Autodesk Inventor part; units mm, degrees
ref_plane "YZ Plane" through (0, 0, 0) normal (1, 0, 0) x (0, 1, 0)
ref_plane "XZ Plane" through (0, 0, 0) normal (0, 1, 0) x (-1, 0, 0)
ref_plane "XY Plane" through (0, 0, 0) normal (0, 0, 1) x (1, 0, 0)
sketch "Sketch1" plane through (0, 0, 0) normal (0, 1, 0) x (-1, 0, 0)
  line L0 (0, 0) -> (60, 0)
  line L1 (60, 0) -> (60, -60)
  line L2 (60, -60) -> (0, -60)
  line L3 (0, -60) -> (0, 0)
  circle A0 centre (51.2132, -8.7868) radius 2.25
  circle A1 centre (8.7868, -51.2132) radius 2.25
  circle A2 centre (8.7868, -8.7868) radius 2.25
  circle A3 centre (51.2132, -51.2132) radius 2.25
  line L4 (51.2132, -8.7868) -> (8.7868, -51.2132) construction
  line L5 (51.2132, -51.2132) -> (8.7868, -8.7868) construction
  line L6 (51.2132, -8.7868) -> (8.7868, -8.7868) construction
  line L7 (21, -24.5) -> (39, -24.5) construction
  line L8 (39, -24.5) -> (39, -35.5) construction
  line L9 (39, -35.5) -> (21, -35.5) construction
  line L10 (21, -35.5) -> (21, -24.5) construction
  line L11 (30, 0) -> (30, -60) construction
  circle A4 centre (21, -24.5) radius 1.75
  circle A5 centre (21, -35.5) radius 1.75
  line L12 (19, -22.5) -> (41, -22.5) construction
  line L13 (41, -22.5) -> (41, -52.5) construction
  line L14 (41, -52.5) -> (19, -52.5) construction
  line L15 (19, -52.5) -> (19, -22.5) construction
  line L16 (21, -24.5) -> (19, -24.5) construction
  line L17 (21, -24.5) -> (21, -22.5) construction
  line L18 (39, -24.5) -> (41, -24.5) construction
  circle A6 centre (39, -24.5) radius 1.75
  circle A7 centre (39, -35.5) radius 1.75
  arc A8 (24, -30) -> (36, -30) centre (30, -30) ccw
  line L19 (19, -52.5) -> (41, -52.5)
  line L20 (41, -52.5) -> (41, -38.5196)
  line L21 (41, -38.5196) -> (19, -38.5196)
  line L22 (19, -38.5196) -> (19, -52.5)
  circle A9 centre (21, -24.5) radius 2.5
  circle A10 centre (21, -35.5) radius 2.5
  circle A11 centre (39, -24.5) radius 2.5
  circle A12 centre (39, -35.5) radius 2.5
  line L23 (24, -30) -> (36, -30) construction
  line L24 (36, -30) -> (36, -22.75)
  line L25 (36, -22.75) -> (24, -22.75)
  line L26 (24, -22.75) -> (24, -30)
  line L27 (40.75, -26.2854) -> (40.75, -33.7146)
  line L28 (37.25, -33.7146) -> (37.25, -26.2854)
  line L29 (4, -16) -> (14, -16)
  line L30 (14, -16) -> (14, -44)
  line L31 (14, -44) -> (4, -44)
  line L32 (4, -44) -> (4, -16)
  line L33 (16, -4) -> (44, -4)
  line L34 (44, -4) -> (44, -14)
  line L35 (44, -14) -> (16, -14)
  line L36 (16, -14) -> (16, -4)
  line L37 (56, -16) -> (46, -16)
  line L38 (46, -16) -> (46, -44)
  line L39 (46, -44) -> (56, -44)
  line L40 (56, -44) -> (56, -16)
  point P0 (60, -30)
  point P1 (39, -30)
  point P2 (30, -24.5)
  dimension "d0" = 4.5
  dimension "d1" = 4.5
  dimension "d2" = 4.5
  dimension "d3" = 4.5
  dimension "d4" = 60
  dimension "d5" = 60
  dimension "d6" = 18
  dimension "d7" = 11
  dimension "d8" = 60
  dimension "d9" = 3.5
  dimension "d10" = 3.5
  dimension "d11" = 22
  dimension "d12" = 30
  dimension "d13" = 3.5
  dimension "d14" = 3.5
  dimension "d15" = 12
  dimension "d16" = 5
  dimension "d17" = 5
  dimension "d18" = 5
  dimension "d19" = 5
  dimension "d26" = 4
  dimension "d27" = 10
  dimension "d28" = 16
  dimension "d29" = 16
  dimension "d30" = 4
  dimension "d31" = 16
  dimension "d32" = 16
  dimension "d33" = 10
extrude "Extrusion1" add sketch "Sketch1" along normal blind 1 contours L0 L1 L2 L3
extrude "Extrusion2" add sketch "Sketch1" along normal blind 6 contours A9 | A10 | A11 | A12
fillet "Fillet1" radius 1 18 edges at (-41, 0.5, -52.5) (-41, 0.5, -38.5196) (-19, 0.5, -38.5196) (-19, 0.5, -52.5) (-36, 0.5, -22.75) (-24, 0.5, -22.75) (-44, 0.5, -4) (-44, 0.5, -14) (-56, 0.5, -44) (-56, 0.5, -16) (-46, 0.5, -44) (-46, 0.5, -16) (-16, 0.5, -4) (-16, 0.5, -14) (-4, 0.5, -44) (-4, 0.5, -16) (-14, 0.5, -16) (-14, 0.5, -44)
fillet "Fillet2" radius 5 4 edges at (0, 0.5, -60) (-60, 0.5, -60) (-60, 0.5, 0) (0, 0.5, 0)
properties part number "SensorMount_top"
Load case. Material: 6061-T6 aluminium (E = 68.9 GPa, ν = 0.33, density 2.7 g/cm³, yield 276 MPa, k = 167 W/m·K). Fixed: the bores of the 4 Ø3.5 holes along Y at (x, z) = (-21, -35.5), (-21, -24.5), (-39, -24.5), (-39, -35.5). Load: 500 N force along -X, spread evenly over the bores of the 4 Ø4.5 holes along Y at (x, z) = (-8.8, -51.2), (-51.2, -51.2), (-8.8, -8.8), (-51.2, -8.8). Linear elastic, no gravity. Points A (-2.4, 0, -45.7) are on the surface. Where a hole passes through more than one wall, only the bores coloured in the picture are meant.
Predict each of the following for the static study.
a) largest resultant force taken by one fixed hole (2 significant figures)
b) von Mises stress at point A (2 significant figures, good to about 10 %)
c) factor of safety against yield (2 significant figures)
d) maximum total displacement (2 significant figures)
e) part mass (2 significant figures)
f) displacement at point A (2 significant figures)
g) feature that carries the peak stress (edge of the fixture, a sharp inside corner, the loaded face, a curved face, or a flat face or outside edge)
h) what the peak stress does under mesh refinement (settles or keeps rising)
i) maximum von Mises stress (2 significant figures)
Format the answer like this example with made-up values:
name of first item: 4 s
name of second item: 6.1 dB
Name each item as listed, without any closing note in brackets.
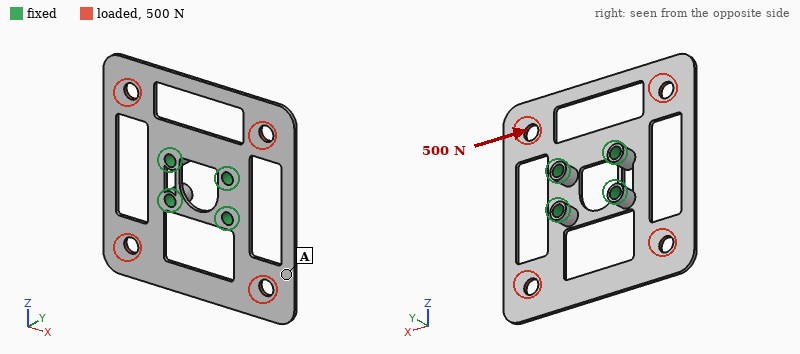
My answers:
largest resultant force taken by one fixed hole: 180 N
von Mises stress at point A: 14 MPa
factor of safety against yield: 1.1
maximum total displacement: 42 µm
part mass: 6.4 g
displacement at point A: 31 µm
feature that carries the peak stress: a curved face
what the peak stress does under mesh refinement: settles
maximum von Mises stress: 250 MPa
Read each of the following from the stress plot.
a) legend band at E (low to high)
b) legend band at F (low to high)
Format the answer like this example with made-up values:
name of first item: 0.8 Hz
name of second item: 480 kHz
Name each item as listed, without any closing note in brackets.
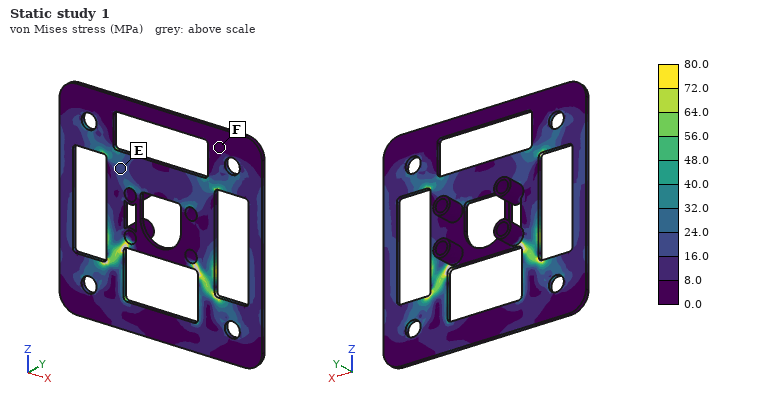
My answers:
legend band at E: 16.0 to 24.0 MPa
legend band at F: 0.0 to 8.0 MPa
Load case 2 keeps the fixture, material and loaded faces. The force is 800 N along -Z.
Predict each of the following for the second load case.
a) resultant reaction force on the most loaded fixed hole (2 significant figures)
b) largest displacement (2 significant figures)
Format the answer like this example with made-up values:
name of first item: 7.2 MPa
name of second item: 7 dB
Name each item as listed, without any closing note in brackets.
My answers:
resultant reaction force on the most loaded fixed hole: 220 N
largest displacement: 24 µm
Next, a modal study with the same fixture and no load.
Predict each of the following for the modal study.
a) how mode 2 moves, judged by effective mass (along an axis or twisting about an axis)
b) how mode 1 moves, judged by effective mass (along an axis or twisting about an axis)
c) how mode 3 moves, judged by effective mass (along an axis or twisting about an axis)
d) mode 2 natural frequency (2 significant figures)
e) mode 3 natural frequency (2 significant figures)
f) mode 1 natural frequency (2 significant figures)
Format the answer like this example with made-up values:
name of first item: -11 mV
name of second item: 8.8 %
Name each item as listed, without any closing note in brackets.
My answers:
how mode 2 moves, judged by effective mass: twisting about Z
how mode 1 moves, judged by effective mass: along Y
how mode 3 moves, judged by effective mass: along Y
mode 2 natural frequency: 850 Hz
mode 3 natural frequency: 890 Hz
mode 1 natural frequency: 720 Hz
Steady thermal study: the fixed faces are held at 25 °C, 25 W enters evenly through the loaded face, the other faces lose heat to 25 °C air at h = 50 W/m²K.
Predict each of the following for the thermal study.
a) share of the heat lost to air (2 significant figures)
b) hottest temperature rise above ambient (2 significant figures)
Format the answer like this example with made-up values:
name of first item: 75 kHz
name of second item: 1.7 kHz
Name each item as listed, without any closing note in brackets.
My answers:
share of the heat lost to air: 41 %
hottest temperature rise above ambient: 67 K
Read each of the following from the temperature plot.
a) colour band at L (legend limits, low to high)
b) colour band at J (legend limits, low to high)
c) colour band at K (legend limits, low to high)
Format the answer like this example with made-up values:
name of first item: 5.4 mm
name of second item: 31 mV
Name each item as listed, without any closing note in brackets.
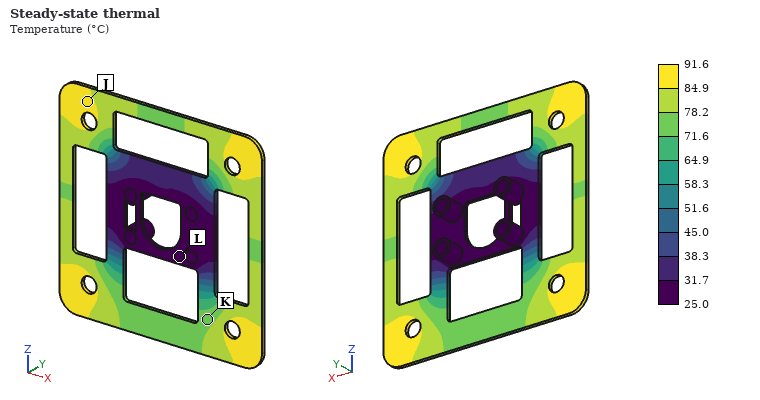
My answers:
colour band at L: 25.0 to 31.7 °C
colour band at J: 84.9 to 91.6 °C
colour band at K: 71.6 to 78.2 °C
